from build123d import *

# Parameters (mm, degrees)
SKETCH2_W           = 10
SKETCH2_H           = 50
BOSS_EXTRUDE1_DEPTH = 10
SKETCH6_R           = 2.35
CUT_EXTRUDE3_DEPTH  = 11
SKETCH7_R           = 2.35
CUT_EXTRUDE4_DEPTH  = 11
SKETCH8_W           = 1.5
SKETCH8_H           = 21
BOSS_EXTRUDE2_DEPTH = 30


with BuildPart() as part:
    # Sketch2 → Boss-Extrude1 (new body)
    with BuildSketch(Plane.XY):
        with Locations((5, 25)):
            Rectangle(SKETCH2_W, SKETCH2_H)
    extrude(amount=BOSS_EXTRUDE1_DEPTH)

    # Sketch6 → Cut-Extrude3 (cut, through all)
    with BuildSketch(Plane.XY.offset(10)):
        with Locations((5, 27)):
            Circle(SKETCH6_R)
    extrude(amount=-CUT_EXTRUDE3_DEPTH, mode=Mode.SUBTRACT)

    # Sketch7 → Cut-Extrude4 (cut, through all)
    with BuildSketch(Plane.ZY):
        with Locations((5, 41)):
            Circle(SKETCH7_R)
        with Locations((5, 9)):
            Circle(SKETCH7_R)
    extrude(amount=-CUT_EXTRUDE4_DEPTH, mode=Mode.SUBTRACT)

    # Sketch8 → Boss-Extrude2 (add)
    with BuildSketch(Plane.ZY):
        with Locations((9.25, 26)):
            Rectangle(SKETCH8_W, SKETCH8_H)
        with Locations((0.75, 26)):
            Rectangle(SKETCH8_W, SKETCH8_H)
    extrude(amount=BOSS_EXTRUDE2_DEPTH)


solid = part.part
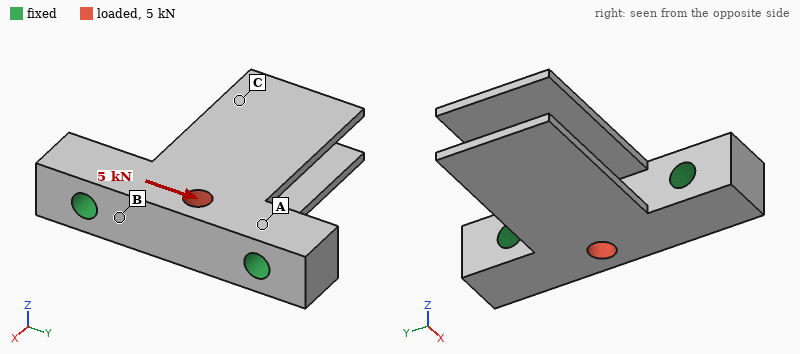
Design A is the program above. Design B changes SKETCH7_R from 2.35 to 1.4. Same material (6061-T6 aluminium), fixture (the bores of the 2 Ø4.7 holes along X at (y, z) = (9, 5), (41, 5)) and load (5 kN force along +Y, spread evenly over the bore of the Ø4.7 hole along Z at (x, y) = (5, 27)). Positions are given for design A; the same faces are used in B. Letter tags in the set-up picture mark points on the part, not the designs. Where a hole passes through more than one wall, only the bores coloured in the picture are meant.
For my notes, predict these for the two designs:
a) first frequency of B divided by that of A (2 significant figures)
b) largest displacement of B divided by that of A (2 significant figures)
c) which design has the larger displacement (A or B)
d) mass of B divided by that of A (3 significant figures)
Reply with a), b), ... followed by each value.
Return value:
a) 1.0
b) 1.1
c) B
d) 1.04
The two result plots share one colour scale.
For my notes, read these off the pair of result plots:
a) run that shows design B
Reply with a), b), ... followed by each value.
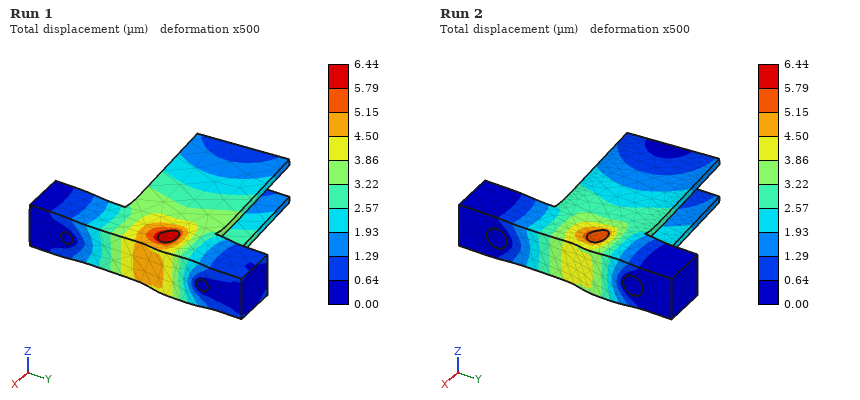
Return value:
a) Run 1
